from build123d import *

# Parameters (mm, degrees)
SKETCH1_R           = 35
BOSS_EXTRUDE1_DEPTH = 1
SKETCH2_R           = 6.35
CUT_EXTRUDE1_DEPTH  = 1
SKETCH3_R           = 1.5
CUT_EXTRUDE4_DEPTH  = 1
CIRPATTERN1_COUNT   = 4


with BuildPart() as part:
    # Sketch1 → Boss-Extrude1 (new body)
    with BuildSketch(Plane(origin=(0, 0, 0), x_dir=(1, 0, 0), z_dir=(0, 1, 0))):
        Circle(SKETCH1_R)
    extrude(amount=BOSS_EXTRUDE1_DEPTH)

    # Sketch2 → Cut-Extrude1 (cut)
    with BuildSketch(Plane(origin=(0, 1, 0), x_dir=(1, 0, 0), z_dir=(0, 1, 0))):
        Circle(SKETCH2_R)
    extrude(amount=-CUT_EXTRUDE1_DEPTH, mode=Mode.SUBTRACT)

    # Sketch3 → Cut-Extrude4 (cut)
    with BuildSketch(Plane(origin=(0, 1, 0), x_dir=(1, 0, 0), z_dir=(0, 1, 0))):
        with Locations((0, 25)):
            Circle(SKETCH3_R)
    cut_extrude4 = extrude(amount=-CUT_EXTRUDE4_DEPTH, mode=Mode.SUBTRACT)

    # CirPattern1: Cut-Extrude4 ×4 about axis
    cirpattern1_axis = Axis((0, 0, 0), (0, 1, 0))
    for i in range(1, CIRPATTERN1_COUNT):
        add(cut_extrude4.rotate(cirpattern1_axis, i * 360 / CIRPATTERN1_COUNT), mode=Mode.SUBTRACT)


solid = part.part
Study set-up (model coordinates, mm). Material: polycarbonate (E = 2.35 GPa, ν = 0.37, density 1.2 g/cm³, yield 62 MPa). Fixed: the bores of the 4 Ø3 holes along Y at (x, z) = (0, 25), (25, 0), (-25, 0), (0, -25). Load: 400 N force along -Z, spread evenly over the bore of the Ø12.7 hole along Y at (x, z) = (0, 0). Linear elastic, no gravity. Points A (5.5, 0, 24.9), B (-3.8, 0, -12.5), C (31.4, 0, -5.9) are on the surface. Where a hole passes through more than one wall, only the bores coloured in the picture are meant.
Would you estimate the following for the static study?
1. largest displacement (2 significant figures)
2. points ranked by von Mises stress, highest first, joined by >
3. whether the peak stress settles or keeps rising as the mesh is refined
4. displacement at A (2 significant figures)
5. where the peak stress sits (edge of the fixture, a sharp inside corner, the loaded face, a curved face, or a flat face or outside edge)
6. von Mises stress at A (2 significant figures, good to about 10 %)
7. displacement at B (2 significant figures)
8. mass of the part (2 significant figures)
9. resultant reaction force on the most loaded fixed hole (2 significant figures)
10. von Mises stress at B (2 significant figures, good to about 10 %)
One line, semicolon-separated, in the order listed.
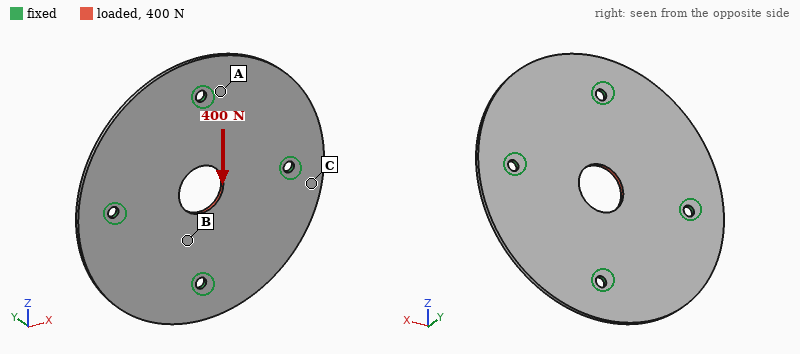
92 µm; B > A > C; keeps rising; 24 µm; edge of the fixture; 4.6 MPa; 57 µm; 4.4 g; 130 N; 9.1 MPa
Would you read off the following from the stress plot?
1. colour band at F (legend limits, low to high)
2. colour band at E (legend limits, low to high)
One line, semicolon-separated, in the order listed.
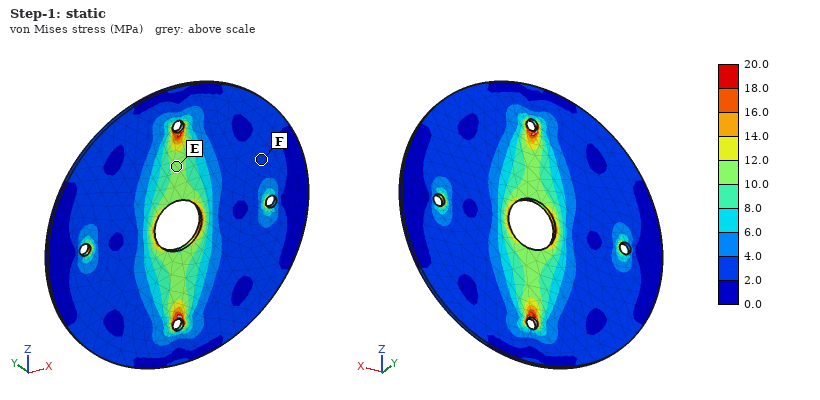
2.0 to 4.0 MPa; 10.0 to 12.0 MPa
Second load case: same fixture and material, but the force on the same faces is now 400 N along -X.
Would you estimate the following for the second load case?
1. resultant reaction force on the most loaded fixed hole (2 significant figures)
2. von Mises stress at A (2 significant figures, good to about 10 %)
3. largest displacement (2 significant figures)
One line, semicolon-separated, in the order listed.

130 N; 4.3 MPa; 92 µm
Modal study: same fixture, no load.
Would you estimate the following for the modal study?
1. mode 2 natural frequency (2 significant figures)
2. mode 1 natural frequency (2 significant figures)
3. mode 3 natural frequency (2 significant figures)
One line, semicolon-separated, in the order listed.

730 Hz; 690 Hz; 730 Hz
